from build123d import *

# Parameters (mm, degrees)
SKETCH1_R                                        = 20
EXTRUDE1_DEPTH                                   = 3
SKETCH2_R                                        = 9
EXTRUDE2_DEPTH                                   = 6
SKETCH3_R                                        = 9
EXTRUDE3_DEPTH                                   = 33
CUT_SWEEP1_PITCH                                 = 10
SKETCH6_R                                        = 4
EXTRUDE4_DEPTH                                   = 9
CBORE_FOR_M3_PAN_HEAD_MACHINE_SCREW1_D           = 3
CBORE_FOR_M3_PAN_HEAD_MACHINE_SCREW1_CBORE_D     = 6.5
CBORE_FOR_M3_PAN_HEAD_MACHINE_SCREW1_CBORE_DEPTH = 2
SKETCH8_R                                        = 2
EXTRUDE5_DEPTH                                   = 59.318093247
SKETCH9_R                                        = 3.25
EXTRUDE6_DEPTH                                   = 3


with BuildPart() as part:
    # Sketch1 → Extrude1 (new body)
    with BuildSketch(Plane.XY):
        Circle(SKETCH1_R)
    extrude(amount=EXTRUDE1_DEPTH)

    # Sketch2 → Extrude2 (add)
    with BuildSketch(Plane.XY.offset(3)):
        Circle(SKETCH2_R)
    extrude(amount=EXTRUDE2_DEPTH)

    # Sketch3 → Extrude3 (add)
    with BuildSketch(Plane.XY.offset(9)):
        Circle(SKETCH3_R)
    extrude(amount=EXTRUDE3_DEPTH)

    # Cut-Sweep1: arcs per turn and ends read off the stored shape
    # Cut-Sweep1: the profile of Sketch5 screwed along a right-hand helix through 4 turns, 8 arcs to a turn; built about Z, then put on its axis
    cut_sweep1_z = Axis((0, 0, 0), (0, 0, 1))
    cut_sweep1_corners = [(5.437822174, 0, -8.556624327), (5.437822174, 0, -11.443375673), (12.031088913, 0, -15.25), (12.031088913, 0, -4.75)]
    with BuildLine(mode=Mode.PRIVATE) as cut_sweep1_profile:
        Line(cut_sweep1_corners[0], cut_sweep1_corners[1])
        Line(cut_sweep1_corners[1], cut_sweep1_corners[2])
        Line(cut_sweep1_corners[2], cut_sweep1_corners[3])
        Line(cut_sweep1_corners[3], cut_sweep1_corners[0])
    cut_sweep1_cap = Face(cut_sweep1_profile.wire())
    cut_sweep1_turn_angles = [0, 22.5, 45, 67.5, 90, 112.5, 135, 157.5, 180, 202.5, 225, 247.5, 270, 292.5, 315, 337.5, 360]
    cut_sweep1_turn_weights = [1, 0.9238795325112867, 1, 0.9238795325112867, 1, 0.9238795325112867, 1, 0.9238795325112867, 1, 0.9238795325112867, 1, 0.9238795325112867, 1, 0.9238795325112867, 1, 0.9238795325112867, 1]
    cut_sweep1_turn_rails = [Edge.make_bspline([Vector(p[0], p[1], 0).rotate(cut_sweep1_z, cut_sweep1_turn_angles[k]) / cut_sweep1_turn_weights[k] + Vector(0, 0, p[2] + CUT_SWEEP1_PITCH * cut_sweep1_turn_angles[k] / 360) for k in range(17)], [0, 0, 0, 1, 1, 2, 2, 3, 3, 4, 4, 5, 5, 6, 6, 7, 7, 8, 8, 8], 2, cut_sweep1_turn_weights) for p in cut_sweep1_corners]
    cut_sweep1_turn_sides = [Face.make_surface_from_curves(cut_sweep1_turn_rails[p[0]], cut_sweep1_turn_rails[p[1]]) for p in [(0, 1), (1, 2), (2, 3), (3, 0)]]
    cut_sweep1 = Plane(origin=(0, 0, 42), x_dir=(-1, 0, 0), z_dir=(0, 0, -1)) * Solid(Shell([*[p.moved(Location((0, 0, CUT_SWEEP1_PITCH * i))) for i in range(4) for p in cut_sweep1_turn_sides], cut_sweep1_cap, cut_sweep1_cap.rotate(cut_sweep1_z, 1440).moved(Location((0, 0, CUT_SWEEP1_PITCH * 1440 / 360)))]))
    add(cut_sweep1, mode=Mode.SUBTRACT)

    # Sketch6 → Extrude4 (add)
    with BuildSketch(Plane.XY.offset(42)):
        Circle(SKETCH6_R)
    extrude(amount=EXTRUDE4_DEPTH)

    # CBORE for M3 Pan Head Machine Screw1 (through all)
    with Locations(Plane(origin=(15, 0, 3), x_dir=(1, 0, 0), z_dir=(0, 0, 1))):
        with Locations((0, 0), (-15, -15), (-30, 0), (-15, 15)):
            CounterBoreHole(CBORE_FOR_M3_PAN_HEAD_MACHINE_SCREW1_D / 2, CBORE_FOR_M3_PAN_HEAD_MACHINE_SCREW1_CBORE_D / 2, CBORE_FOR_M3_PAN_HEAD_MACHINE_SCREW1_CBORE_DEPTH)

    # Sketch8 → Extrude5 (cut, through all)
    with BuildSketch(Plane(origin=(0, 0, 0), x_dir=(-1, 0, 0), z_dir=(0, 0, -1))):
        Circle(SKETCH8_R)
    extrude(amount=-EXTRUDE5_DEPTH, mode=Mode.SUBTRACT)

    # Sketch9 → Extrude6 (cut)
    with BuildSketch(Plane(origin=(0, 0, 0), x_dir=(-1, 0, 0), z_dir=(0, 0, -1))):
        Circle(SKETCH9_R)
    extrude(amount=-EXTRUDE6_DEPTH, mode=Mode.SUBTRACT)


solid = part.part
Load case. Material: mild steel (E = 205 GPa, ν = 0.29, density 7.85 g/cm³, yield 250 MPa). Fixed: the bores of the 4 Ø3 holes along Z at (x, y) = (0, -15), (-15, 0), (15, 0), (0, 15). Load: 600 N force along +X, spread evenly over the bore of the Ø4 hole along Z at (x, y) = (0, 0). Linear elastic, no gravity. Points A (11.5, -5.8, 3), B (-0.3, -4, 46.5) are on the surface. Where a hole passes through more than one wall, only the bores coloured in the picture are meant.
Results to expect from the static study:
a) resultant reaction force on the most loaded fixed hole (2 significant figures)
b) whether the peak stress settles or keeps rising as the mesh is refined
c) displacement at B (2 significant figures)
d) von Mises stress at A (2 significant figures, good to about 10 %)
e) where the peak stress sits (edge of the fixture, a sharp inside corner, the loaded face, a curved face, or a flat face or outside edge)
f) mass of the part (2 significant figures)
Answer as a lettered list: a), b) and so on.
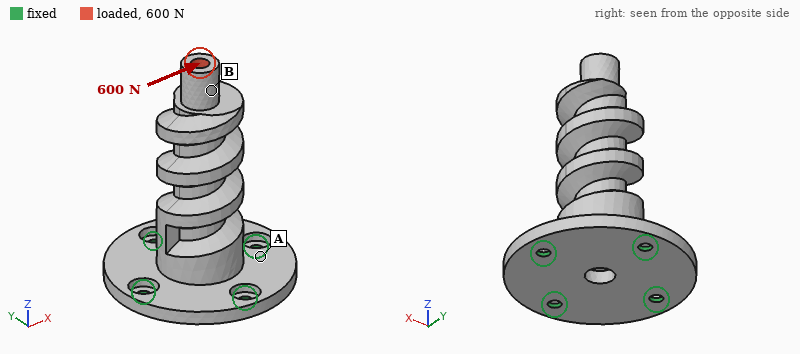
a) 690 N
b) keeps rising
c) 52 µm
d) 38 MPa
e) edge of the fixture
f) 84 g
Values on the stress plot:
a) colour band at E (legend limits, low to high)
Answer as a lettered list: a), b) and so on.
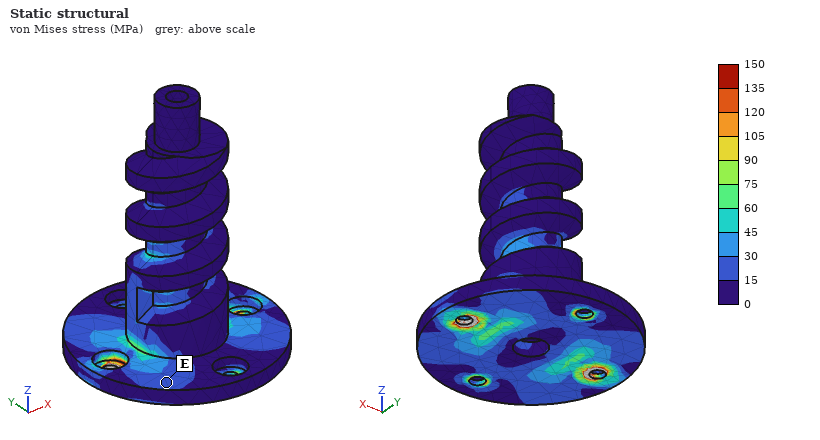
a) 15 to 30 MPa
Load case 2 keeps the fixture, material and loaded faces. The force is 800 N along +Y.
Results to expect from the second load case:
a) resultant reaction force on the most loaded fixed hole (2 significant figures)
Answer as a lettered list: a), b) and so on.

a) 930 N
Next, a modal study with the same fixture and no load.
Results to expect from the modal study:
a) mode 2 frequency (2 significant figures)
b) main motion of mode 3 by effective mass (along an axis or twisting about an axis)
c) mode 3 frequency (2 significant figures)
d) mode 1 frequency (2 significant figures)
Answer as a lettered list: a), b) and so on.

a) 3300 Hz
b) along Z
c) 9100 Hz
d) 3200 Hz
